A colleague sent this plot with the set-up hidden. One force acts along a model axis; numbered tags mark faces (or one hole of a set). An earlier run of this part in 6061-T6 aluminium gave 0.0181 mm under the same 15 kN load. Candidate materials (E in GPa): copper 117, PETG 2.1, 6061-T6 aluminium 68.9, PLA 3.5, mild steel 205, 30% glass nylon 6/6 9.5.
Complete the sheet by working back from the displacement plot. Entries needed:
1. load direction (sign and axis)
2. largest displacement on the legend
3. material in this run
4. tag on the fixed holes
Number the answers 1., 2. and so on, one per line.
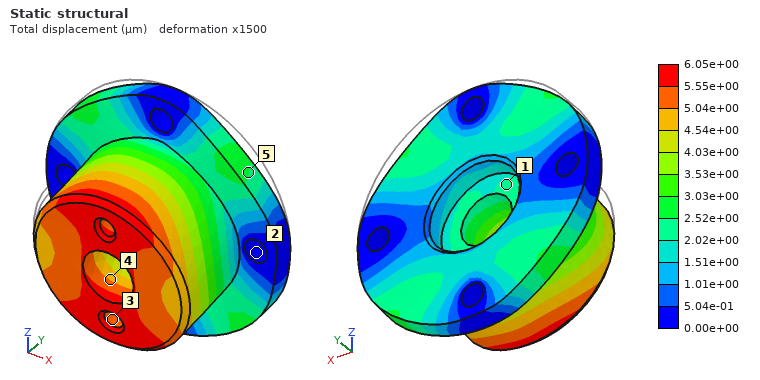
1. -Z
2. 6.05e+00 µm
3. mild steel
4. 2
